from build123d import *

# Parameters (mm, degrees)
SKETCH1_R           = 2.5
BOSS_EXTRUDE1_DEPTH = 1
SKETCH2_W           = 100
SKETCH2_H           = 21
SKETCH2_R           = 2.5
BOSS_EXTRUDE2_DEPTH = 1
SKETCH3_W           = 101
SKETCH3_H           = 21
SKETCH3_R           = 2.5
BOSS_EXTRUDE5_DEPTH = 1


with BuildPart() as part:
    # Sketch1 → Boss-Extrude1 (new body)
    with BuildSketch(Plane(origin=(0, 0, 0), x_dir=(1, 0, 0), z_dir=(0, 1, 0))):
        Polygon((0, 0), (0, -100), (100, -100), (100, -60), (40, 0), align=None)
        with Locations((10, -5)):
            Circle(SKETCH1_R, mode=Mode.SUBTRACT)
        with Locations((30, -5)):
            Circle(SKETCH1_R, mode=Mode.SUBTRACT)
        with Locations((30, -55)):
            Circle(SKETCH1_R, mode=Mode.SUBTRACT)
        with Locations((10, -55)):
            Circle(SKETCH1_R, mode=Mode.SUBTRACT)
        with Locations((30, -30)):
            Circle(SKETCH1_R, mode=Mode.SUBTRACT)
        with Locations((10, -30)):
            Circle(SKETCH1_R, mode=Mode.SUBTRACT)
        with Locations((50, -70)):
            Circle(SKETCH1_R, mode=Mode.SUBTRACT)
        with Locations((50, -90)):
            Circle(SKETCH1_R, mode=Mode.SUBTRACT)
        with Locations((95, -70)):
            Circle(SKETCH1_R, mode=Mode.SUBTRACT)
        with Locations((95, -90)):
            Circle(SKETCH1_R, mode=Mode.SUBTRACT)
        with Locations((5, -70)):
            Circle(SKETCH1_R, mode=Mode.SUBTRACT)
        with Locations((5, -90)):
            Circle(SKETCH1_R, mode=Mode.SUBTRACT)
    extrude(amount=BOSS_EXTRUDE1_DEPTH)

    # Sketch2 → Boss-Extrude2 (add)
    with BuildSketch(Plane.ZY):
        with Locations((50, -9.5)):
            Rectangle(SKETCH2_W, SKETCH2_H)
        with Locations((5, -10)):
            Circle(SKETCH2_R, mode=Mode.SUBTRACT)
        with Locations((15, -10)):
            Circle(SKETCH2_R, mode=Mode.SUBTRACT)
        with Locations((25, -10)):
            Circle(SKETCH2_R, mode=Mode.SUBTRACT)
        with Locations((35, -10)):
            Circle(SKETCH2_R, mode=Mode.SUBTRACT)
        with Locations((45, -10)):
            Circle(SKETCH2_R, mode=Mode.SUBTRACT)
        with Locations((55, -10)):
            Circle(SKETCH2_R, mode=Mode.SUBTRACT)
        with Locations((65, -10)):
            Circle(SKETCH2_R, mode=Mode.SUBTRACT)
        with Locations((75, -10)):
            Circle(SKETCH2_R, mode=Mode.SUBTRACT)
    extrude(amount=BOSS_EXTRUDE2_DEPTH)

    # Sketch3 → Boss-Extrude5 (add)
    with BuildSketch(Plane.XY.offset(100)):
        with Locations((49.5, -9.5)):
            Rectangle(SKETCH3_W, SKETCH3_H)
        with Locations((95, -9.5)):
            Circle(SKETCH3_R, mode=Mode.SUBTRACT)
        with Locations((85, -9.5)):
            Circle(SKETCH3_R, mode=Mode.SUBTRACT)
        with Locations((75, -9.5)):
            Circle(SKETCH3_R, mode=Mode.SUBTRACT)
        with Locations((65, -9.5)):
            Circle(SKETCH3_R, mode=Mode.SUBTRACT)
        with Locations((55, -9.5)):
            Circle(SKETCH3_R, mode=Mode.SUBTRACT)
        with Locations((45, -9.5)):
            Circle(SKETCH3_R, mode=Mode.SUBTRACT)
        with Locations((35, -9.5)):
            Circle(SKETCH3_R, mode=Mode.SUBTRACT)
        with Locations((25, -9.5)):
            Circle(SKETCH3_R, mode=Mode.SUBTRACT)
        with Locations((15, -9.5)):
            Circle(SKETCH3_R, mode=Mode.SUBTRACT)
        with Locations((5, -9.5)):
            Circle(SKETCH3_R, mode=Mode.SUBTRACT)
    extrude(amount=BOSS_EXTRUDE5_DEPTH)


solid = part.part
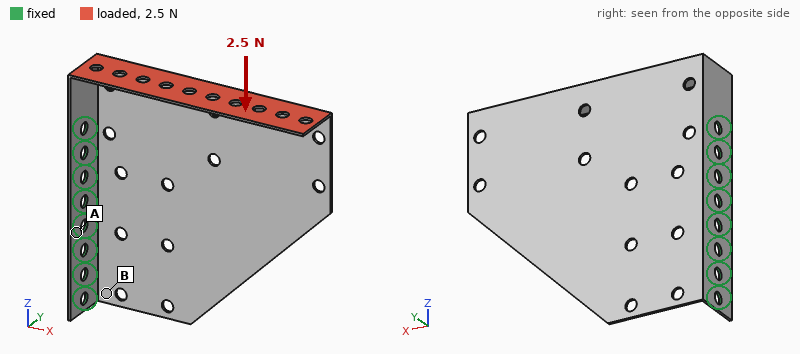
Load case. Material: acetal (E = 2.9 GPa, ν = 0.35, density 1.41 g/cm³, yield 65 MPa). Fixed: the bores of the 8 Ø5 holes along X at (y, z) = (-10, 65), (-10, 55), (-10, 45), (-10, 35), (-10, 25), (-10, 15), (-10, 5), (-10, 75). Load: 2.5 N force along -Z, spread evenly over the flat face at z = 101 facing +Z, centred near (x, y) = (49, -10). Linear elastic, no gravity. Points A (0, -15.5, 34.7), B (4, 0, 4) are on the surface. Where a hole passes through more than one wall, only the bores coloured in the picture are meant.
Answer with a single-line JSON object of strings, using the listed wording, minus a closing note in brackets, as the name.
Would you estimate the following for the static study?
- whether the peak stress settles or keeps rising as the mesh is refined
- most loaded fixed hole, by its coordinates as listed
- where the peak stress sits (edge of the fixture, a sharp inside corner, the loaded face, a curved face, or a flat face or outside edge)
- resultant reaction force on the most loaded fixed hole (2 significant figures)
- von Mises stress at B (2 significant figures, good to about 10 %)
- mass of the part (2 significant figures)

{"whether the peak stress settles or keeps rising as the mesh is refined": "keeps rising", "most loaded fixed hole, by its coordinates as listed": "(-10, 75)", "where the peak stress sits": "edge of the fixture", "resultant reaction force on the most loaded fixed hole": "1.4 N", "von Mises stress at B": "0.47 MPa", "mass of the part": "17 g"}
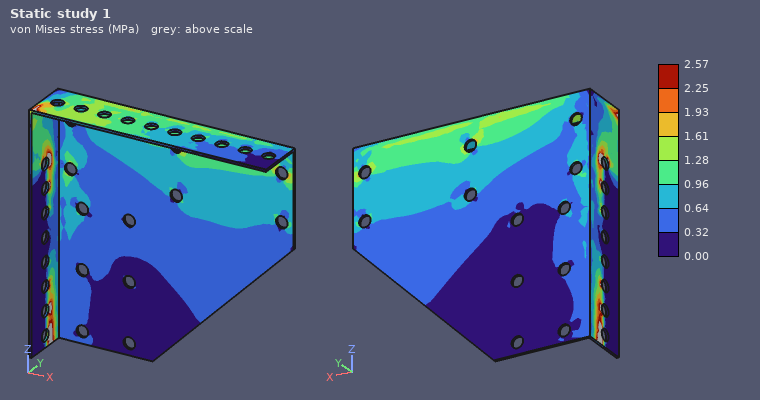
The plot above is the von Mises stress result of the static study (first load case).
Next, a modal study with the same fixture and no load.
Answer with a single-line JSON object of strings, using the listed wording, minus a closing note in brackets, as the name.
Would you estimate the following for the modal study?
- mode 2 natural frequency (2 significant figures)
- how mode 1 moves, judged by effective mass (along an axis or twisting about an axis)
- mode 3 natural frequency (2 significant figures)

{"mode 2 natural frequency": "73 Hz", "how mode 1 moves, judged by effective mass": "along Y", "mode 3 natural frequency": "170 Hz"}
